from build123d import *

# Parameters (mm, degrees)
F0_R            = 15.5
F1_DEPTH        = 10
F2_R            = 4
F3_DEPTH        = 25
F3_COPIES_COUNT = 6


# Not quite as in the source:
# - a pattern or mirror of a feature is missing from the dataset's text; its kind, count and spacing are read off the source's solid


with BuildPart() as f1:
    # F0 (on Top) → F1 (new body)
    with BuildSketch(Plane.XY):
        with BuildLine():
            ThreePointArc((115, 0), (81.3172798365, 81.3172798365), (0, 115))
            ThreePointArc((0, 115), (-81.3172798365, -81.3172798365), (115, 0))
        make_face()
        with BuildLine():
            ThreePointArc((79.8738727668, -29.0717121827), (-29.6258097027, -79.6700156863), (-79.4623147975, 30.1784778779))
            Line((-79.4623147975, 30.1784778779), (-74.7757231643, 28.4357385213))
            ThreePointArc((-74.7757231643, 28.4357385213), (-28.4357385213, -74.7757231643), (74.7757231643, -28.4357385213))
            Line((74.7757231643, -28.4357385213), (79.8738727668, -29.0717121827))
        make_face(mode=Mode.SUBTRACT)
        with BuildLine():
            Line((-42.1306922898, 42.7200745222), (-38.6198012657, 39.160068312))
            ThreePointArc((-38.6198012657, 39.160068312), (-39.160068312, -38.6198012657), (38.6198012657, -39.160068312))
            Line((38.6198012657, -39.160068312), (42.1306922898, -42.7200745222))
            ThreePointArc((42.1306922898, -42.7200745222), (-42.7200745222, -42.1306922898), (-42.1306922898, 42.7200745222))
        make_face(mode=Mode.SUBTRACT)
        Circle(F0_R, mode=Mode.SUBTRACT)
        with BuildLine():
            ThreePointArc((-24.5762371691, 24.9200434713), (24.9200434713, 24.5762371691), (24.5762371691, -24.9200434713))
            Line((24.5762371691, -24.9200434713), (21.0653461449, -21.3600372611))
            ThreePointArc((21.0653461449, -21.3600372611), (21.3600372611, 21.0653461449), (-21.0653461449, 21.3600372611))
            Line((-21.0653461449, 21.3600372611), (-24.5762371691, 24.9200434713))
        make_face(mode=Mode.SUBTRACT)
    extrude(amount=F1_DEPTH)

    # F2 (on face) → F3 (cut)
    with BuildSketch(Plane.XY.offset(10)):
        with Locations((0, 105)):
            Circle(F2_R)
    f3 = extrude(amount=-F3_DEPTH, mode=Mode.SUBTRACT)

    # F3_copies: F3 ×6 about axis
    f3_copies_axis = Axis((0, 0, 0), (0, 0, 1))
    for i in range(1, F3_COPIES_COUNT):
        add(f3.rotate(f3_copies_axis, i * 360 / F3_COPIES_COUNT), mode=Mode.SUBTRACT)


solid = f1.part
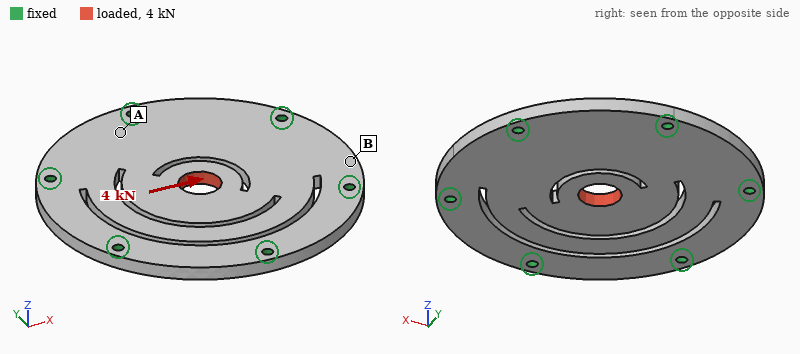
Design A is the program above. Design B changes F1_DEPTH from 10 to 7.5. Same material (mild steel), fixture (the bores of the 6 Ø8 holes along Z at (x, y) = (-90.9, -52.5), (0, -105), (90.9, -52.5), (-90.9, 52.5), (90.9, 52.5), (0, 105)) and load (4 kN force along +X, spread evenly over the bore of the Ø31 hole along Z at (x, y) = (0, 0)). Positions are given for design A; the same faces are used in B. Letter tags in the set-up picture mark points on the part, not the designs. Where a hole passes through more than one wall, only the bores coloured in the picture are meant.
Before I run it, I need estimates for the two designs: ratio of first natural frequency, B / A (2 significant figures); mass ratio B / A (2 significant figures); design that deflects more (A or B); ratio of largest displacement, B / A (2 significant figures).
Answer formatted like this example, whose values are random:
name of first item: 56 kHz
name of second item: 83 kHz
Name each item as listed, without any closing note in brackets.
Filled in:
ratio of first natural frequency, B / A: 0.77
mass ratio B / A: 0.75
design that deflects more: B
ratio of largest displacement, B / A: 1.3
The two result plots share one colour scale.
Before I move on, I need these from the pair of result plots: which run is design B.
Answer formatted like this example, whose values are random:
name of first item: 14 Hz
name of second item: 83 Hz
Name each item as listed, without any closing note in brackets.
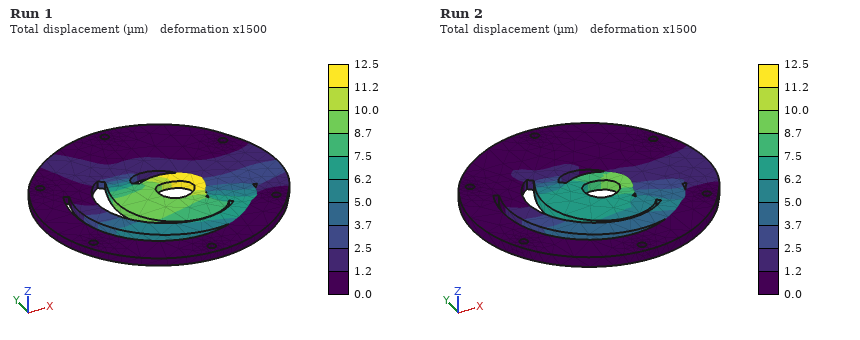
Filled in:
which run is design B: Run 1
